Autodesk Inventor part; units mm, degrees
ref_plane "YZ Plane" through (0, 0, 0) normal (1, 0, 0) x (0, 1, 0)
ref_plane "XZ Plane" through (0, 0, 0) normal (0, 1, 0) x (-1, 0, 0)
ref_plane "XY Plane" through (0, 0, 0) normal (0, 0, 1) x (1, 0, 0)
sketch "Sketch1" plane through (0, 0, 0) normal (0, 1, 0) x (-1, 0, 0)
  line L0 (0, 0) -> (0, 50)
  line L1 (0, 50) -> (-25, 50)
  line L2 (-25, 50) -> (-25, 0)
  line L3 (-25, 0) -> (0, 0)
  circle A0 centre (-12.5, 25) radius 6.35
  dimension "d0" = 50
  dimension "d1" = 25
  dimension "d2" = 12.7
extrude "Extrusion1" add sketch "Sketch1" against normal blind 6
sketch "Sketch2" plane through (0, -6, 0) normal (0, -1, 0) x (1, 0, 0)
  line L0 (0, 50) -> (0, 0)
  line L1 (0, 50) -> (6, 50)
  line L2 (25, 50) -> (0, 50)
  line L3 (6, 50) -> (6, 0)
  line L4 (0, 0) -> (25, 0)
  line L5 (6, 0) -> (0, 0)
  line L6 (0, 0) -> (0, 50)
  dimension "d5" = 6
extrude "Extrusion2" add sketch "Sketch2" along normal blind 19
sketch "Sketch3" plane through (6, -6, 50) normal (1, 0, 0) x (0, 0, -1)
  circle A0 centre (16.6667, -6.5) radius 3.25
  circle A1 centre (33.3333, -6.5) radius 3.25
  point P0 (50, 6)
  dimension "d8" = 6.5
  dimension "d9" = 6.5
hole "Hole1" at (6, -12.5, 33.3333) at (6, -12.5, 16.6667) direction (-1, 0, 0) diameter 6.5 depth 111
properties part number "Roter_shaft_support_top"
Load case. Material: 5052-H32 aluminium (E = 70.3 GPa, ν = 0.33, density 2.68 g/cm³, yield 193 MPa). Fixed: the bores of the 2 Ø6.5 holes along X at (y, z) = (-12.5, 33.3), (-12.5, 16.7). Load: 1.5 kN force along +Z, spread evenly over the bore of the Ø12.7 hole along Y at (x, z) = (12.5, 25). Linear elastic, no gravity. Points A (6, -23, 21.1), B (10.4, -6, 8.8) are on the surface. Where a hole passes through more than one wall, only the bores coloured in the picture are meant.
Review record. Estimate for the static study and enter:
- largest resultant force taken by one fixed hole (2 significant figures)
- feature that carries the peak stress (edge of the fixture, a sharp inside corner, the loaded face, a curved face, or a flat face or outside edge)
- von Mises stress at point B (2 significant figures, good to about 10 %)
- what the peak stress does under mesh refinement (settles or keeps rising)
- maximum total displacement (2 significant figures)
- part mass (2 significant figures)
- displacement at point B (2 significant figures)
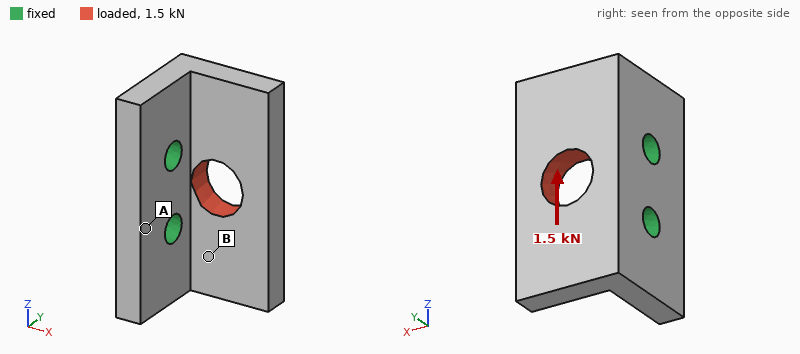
1.0 kN
edge of the fixture
12 MPa
keeps rising
24 µm
32 g
10 µm
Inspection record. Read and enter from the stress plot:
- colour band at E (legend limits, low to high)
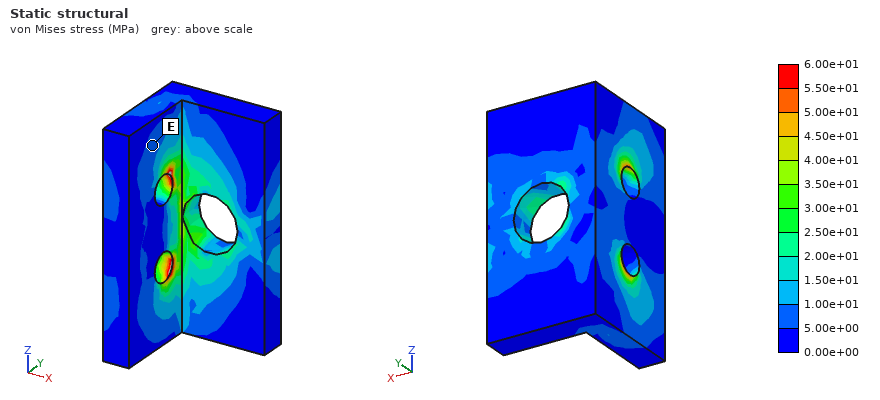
5.00e+00 to 1.00e+01 MPa
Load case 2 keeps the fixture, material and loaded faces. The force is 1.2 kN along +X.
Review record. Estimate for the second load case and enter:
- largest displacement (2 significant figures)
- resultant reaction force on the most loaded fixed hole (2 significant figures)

20 µm
600 N
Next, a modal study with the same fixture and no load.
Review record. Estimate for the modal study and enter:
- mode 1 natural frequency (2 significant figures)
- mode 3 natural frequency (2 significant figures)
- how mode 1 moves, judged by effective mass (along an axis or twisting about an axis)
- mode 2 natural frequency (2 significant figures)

6300 Hz
12 kHz
along Y
8400 Hz
